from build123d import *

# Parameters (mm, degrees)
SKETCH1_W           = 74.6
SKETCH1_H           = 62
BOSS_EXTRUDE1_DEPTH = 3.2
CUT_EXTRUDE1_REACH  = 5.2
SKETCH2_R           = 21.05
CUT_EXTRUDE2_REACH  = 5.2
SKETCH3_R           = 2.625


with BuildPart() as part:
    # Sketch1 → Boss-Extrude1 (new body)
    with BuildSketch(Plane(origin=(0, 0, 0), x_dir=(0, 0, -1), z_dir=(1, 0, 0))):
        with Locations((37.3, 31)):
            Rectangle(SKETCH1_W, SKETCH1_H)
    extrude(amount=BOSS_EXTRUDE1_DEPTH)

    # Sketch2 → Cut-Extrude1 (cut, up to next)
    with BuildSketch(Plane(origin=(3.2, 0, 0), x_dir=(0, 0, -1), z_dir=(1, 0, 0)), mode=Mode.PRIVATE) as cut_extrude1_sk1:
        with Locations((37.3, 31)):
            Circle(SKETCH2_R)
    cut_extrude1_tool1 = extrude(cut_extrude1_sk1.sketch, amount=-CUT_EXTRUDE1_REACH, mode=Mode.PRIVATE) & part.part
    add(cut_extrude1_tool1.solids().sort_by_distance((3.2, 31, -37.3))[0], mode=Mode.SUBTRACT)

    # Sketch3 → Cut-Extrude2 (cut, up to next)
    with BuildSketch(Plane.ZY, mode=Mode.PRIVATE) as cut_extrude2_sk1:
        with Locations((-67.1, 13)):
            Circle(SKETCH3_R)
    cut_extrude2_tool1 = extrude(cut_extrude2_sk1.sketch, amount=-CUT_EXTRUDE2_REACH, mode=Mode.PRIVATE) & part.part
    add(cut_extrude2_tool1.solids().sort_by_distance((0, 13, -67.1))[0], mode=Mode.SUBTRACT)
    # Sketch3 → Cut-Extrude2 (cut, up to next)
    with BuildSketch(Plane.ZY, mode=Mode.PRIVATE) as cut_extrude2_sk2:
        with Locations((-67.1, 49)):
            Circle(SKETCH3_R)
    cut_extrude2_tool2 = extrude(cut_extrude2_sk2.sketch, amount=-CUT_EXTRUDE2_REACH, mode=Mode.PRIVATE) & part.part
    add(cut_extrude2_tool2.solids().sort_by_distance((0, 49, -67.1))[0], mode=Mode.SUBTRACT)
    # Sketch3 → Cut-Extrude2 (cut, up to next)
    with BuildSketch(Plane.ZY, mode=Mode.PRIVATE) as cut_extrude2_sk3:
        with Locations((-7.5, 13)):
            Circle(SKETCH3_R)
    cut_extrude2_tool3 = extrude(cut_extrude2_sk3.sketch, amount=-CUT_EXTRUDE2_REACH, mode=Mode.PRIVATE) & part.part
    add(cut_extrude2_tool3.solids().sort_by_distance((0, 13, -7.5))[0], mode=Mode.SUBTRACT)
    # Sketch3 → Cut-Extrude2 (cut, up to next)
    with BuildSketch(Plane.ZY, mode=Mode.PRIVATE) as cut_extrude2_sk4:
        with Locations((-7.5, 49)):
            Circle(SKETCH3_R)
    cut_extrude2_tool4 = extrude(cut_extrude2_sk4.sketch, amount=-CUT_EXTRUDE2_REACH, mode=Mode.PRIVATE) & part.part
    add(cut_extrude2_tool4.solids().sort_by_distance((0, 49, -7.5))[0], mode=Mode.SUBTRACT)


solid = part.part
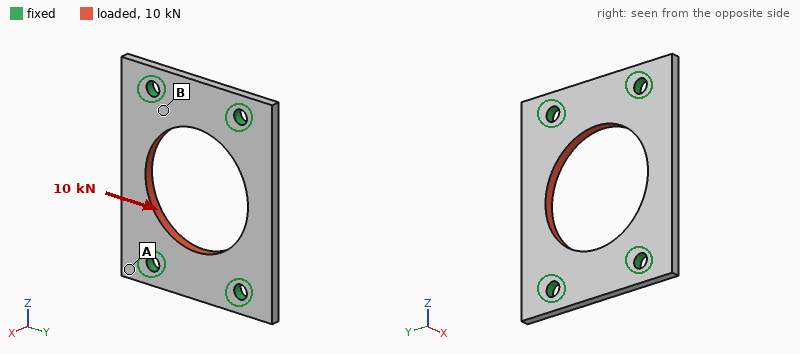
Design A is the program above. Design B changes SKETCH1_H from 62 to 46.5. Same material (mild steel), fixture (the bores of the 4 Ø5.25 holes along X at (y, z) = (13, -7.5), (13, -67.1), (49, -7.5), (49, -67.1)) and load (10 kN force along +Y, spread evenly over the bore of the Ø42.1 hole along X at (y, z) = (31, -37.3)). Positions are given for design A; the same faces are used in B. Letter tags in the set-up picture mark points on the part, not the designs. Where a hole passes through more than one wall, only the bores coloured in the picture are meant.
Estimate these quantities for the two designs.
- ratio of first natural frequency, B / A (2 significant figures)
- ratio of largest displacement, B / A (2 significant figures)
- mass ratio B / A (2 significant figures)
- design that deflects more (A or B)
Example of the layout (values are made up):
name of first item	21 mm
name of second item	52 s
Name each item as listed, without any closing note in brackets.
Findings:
ratio of first natural frequency, B / A	1.4
ratio of largest displacement, B / A	3.7
mass ratio B / A	0.63
design that deflects more	B
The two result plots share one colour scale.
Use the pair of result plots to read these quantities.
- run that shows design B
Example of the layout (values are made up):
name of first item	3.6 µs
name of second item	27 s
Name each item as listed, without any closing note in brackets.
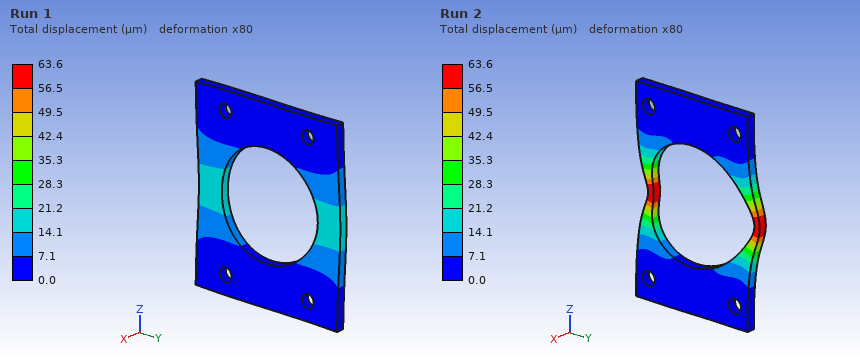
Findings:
run that shows design B	Run 2
